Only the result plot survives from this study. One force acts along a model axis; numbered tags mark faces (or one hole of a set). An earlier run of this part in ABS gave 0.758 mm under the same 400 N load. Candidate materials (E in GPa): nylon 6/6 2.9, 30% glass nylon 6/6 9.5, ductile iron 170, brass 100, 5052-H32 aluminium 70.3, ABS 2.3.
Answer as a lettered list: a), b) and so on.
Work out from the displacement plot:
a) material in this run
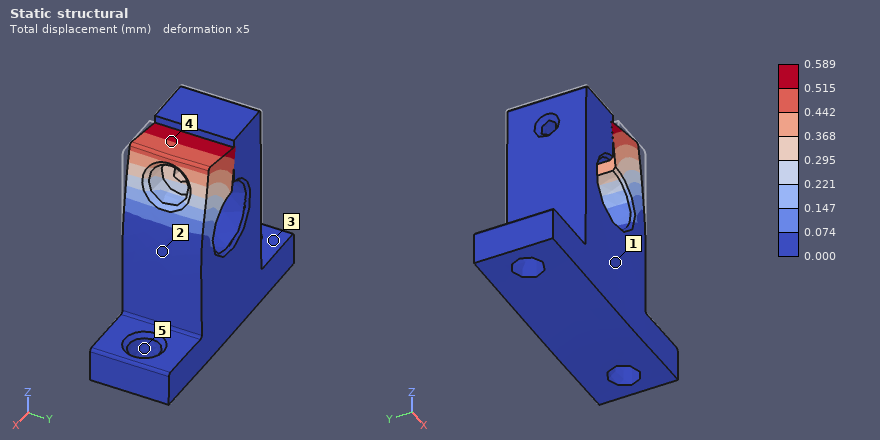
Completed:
a) nylon 6/6
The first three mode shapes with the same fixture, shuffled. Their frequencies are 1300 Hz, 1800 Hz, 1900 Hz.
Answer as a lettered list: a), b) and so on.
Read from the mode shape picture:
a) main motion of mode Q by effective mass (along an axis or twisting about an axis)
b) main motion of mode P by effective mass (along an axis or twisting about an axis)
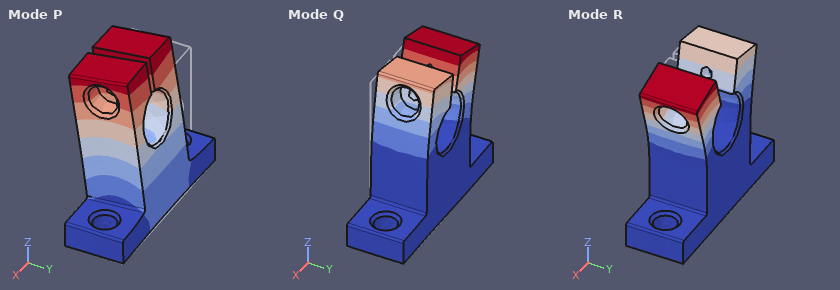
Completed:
a) along X
b) along Y
